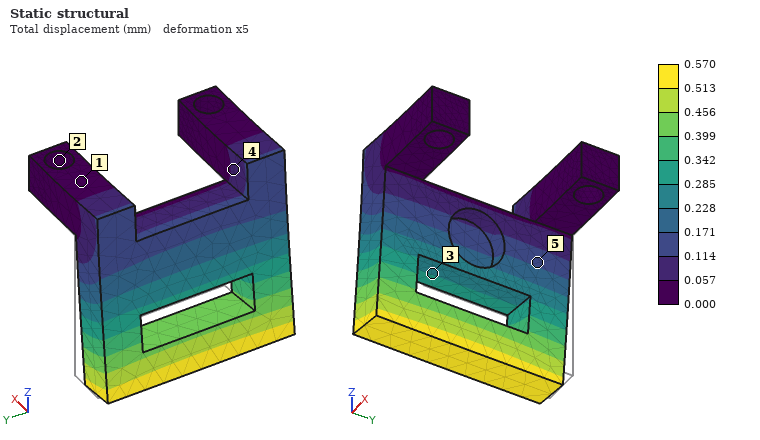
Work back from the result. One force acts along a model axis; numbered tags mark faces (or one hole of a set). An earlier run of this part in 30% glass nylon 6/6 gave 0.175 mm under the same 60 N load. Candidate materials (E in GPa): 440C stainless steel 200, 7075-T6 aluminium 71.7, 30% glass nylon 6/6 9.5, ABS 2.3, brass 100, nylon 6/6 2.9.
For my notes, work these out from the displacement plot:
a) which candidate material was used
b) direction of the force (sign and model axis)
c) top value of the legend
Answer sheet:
nylon 6/6
-X
0.570 mm
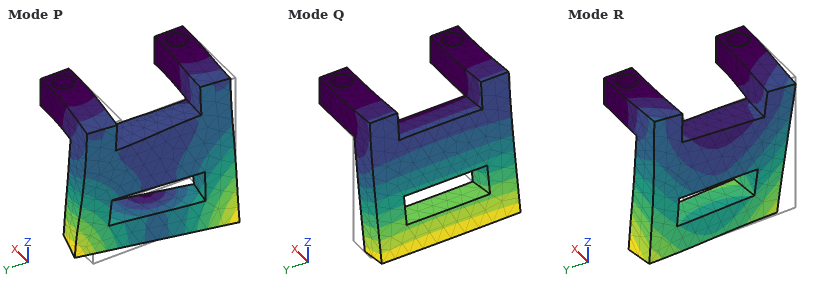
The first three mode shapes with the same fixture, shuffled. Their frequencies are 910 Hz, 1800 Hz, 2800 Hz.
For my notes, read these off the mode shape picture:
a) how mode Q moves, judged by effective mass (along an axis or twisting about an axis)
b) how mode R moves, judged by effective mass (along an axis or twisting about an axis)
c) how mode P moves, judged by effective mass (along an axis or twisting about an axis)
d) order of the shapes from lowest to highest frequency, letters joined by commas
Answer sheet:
along X
along Y
along Y
Q, R, P
